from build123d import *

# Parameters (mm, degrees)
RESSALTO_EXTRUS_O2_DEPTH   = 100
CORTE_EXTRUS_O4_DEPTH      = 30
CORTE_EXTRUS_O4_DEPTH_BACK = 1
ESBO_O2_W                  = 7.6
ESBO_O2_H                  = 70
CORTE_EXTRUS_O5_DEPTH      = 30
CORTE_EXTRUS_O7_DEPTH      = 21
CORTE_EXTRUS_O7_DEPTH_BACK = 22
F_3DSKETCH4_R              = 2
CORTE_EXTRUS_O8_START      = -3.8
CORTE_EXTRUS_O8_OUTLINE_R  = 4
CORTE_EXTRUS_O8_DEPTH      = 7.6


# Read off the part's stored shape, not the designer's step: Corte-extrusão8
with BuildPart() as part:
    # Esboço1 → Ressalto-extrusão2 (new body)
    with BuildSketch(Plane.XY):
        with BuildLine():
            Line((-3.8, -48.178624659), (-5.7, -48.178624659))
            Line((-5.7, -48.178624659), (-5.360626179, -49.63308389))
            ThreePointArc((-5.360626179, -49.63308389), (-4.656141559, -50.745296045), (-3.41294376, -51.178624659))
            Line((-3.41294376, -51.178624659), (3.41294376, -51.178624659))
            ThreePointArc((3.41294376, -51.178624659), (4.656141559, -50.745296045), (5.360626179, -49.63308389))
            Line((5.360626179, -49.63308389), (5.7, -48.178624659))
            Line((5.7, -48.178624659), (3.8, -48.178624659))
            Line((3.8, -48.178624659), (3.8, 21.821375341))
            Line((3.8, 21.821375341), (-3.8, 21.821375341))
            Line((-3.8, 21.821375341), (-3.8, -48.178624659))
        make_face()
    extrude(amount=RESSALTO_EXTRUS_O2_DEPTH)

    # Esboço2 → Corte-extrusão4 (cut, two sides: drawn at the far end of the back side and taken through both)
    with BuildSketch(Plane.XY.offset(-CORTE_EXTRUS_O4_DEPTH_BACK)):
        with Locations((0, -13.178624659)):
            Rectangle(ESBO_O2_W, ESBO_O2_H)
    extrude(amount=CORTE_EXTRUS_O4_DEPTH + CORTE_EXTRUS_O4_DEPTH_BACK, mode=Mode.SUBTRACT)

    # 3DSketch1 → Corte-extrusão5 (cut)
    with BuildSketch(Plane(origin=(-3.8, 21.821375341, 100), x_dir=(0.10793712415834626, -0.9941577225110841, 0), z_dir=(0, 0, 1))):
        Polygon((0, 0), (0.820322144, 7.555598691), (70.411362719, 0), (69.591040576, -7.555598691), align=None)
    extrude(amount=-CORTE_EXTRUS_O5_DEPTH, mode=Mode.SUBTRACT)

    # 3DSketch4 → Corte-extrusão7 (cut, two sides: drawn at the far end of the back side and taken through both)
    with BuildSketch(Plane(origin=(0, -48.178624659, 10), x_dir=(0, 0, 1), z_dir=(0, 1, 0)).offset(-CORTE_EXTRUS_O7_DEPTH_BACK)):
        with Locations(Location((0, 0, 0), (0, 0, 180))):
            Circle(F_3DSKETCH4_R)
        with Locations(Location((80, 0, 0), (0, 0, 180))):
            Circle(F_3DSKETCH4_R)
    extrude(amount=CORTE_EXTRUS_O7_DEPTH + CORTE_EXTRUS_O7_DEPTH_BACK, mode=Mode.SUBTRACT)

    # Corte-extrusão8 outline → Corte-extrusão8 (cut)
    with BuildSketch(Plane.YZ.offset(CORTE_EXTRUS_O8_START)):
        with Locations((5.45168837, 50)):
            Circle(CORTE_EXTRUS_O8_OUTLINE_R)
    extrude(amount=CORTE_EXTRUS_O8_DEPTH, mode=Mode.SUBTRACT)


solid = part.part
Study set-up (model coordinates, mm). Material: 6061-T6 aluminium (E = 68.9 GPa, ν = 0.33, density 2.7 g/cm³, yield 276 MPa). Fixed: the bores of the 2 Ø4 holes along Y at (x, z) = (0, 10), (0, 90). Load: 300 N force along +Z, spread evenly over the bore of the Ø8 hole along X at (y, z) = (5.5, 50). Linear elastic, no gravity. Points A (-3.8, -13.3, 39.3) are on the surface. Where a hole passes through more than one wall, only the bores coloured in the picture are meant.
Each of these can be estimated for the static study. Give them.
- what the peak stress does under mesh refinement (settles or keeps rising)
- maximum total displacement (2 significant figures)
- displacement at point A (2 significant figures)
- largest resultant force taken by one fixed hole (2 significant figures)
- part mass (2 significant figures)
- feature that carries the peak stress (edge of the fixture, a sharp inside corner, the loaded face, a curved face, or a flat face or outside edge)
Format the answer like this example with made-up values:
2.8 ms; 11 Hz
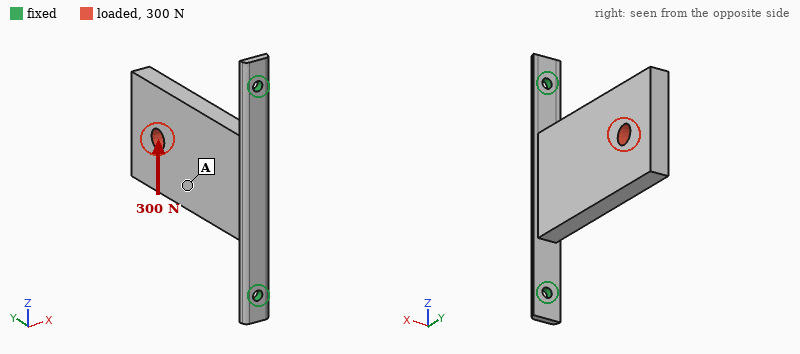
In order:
keeps rising; 0.36 mm; 0.18 mm; 320 N; 65 g; edge of the fixture
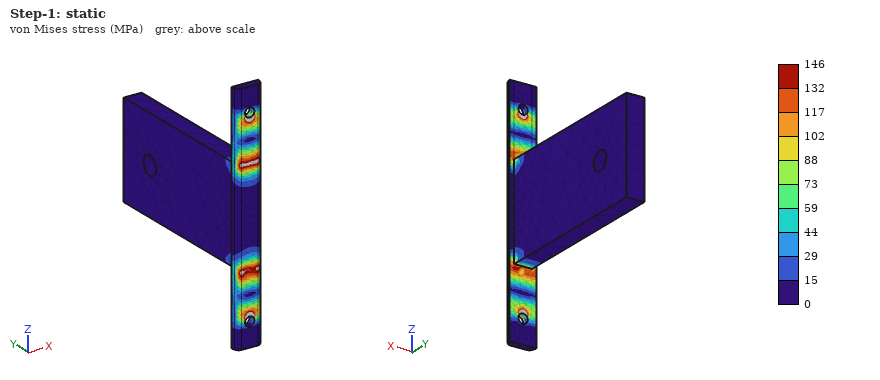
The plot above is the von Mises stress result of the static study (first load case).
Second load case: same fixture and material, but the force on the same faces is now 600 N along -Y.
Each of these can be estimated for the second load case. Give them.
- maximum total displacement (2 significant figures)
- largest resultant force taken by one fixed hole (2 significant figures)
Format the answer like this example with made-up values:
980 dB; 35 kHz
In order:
0.15 mm; 370 N
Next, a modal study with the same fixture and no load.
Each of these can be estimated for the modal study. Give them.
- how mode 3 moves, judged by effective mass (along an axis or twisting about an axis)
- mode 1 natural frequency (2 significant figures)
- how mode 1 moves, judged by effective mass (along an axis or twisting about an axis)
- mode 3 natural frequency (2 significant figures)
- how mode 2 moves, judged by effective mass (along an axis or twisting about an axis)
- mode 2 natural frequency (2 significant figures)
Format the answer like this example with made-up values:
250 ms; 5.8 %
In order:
along Y; 230 Hz; along X; 1300 Hz; along Z; 900 Hz
